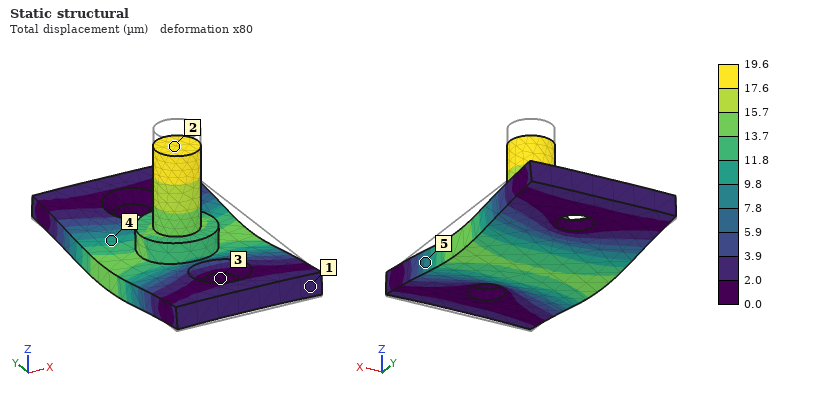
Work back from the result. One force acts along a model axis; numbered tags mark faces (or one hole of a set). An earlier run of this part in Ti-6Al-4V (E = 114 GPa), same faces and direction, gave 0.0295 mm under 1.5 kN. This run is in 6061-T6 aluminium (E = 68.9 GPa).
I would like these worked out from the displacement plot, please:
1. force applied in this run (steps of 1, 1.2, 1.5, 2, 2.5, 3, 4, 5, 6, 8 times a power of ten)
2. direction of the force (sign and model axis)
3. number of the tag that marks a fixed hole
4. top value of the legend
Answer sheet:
600 N
-Z
3
19.6 µm
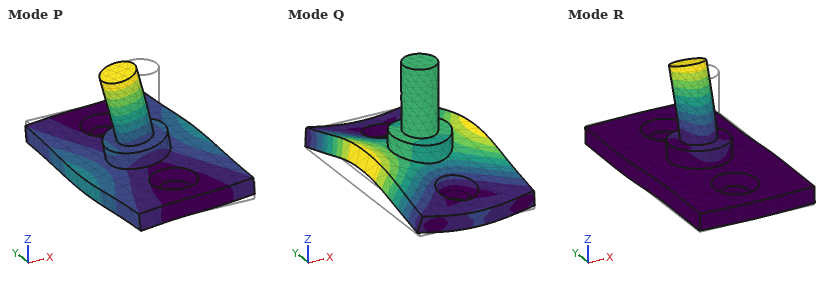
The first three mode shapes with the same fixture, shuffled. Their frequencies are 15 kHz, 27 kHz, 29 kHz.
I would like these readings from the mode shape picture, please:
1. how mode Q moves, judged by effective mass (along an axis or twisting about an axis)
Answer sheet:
along Z
